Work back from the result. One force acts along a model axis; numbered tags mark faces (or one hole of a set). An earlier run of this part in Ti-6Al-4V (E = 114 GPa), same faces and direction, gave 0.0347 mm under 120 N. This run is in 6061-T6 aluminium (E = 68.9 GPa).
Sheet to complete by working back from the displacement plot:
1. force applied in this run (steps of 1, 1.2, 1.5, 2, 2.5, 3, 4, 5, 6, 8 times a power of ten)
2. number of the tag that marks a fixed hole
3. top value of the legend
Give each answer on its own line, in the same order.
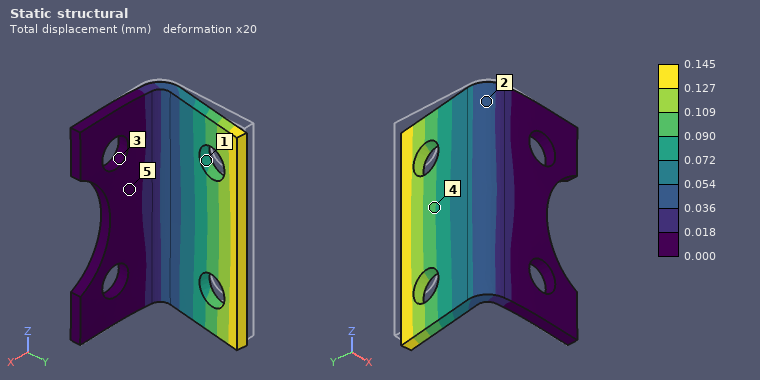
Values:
300 N
3
0.145 mm
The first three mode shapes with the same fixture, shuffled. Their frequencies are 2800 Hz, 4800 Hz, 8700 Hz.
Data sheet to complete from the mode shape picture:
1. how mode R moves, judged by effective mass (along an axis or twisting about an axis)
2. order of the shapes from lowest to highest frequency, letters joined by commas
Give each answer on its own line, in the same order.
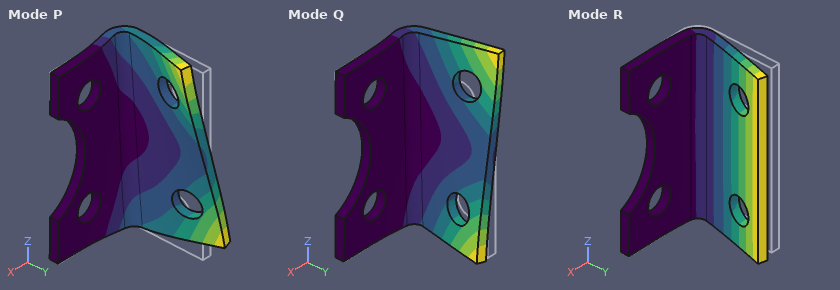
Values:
along X
R, Q, P
